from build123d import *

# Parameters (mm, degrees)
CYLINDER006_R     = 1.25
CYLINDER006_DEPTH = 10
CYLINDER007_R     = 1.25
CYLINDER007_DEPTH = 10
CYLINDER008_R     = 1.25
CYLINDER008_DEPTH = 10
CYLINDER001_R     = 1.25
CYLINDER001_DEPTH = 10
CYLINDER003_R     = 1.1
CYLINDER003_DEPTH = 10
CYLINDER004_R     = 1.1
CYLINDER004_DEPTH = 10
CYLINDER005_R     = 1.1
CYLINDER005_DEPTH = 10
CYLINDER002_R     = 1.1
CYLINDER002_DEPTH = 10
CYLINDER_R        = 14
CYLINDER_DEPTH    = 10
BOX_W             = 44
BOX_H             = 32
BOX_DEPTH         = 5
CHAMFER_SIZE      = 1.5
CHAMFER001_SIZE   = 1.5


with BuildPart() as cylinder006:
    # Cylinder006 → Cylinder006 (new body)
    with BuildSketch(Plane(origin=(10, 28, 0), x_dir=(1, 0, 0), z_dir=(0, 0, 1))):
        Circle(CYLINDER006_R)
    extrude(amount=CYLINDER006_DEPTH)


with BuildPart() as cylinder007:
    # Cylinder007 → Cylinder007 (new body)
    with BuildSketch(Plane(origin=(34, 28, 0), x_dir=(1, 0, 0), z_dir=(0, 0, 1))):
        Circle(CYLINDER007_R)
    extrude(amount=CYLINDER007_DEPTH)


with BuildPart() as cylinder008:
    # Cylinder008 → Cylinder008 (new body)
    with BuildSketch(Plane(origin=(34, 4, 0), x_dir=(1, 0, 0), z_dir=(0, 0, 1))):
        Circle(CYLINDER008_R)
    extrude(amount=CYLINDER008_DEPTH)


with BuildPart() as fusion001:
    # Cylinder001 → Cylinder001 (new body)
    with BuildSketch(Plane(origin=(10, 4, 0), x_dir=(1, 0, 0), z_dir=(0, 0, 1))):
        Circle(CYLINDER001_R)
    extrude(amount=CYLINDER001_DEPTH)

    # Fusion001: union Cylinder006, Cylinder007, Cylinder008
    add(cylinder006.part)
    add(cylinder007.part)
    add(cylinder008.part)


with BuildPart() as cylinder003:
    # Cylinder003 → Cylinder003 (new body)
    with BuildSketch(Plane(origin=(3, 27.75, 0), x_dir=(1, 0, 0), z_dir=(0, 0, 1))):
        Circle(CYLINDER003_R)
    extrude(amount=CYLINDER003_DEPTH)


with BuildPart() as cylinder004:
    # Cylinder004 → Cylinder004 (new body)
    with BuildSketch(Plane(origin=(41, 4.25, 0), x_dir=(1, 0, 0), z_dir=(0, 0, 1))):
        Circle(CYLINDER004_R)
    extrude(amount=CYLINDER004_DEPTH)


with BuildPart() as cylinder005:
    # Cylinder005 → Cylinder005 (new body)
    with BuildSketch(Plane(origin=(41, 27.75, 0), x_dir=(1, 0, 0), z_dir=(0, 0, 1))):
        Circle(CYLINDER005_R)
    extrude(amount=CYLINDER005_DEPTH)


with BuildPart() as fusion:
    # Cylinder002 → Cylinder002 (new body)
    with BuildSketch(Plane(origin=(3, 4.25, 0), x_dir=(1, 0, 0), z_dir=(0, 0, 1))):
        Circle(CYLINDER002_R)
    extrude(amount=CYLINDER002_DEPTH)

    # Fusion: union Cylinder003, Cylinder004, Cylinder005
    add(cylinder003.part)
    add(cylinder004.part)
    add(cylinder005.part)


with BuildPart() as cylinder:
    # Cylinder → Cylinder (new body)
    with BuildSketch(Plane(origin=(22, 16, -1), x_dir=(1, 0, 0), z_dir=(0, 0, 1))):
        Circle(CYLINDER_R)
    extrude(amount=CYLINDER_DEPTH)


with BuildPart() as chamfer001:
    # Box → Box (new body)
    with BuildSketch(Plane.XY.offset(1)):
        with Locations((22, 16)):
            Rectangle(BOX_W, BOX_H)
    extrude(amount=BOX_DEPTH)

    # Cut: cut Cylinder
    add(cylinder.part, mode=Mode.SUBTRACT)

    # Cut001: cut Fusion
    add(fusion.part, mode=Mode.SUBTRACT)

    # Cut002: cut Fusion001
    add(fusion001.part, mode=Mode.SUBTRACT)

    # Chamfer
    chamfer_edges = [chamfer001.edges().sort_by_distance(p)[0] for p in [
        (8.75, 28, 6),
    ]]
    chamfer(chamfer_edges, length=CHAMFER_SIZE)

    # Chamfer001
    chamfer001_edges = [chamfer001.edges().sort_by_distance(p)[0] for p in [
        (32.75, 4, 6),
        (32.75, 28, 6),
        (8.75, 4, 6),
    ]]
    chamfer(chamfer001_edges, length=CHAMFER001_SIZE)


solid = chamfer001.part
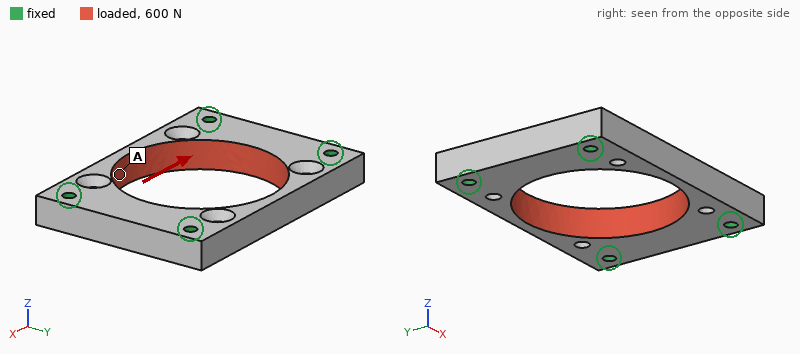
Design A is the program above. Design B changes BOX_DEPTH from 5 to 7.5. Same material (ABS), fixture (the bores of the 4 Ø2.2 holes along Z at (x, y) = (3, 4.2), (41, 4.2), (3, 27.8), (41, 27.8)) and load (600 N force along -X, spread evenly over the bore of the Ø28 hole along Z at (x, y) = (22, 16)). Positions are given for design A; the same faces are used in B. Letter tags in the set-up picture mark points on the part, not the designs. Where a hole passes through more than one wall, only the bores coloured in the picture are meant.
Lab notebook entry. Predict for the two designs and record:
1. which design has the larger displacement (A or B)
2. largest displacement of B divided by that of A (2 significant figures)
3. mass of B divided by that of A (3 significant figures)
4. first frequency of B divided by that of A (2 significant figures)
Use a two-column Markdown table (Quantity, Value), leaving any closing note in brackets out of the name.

| Quantity | Value |
|---|---|
| which design has the larger displacement | A |
| largest displacement of B divided by that of A | 0.67 |
| mass of B divided by that of A | 1.51 |
| first frequency of B divided by that of A | 1.3 |
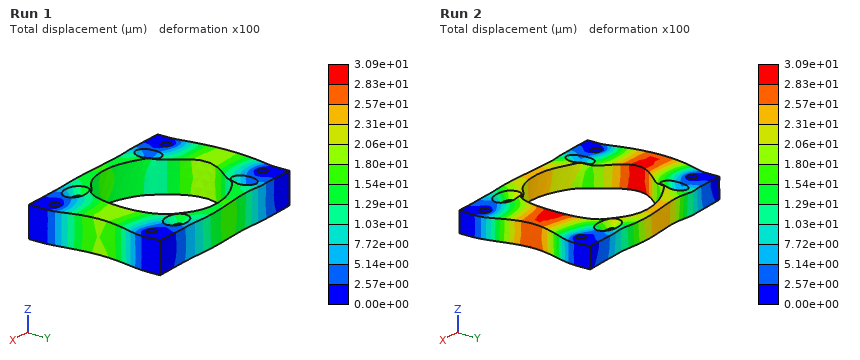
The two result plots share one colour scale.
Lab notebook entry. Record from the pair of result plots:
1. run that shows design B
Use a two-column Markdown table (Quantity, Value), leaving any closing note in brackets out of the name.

| Quantity | Value |
|---|---|
| run that shows design B | Run 1 |
